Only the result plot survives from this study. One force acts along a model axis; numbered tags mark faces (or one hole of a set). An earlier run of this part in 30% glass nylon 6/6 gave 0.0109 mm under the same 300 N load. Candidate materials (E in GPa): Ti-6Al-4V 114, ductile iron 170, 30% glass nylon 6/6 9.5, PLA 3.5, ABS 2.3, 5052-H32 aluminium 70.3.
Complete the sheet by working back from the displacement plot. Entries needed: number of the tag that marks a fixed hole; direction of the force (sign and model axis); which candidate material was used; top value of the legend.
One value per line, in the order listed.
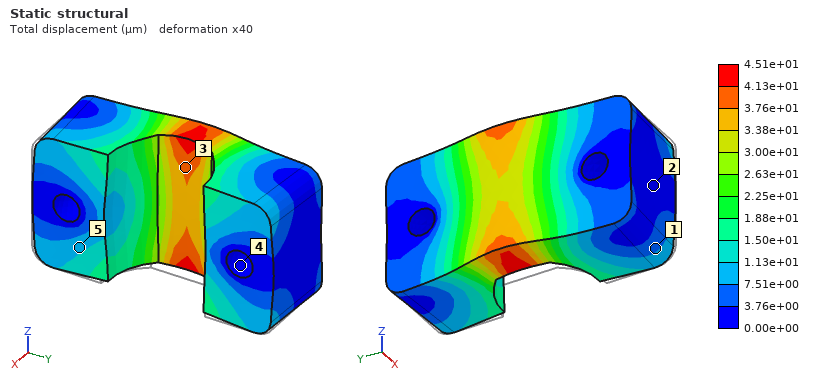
4
-X
ABS
4.51e+01 µm
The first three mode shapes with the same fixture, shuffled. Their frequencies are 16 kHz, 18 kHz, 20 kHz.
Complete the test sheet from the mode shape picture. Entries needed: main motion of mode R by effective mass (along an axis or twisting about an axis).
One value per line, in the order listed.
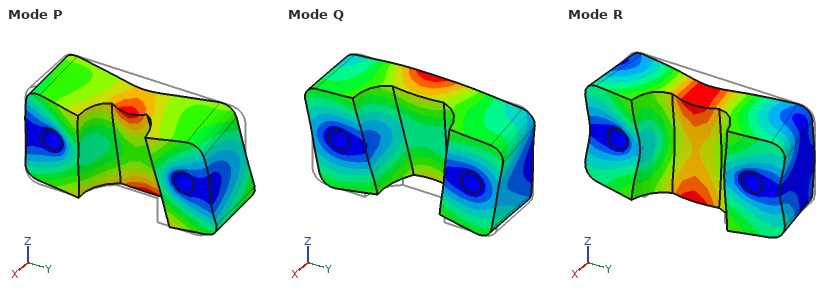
along X
